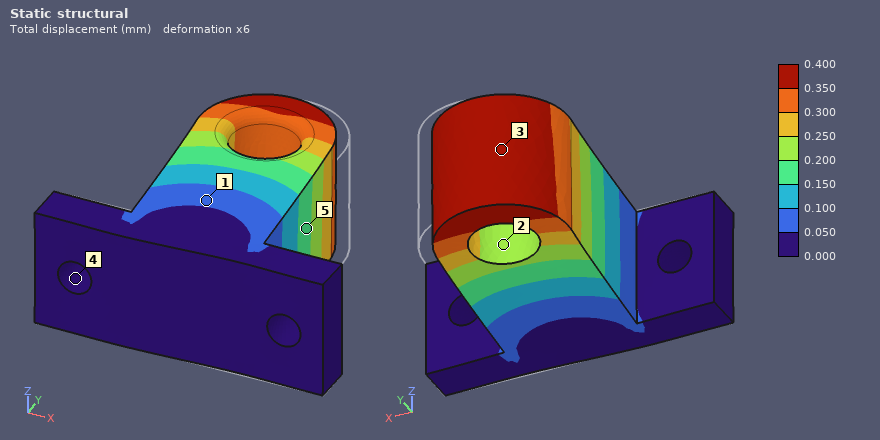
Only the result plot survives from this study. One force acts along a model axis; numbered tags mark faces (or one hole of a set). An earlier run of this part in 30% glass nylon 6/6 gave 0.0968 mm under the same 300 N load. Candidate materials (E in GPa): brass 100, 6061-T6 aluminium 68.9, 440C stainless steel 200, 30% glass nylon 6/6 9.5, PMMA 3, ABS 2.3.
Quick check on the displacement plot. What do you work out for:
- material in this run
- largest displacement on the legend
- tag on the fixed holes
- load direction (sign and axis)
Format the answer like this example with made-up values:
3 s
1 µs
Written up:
ABS
0.400 mm
4
-X
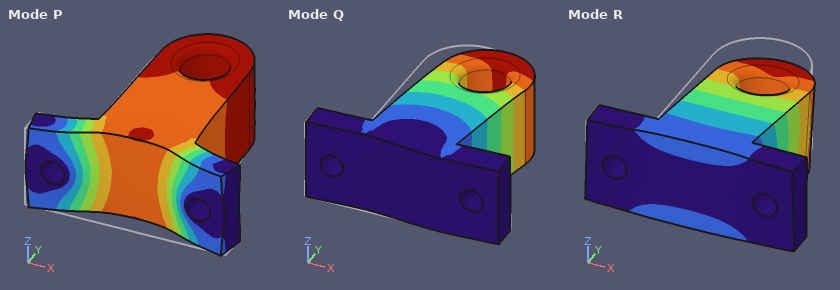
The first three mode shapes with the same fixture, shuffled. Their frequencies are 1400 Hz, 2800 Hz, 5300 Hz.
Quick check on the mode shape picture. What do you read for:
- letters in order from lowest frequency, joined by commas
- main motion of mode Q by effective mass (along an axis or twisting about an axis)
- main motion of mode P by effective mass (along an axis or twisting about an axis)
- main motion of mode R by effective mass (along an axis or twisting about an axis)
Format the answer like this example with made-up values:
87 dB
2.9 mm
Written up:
R, Q, P
along X
along Y
along Z
